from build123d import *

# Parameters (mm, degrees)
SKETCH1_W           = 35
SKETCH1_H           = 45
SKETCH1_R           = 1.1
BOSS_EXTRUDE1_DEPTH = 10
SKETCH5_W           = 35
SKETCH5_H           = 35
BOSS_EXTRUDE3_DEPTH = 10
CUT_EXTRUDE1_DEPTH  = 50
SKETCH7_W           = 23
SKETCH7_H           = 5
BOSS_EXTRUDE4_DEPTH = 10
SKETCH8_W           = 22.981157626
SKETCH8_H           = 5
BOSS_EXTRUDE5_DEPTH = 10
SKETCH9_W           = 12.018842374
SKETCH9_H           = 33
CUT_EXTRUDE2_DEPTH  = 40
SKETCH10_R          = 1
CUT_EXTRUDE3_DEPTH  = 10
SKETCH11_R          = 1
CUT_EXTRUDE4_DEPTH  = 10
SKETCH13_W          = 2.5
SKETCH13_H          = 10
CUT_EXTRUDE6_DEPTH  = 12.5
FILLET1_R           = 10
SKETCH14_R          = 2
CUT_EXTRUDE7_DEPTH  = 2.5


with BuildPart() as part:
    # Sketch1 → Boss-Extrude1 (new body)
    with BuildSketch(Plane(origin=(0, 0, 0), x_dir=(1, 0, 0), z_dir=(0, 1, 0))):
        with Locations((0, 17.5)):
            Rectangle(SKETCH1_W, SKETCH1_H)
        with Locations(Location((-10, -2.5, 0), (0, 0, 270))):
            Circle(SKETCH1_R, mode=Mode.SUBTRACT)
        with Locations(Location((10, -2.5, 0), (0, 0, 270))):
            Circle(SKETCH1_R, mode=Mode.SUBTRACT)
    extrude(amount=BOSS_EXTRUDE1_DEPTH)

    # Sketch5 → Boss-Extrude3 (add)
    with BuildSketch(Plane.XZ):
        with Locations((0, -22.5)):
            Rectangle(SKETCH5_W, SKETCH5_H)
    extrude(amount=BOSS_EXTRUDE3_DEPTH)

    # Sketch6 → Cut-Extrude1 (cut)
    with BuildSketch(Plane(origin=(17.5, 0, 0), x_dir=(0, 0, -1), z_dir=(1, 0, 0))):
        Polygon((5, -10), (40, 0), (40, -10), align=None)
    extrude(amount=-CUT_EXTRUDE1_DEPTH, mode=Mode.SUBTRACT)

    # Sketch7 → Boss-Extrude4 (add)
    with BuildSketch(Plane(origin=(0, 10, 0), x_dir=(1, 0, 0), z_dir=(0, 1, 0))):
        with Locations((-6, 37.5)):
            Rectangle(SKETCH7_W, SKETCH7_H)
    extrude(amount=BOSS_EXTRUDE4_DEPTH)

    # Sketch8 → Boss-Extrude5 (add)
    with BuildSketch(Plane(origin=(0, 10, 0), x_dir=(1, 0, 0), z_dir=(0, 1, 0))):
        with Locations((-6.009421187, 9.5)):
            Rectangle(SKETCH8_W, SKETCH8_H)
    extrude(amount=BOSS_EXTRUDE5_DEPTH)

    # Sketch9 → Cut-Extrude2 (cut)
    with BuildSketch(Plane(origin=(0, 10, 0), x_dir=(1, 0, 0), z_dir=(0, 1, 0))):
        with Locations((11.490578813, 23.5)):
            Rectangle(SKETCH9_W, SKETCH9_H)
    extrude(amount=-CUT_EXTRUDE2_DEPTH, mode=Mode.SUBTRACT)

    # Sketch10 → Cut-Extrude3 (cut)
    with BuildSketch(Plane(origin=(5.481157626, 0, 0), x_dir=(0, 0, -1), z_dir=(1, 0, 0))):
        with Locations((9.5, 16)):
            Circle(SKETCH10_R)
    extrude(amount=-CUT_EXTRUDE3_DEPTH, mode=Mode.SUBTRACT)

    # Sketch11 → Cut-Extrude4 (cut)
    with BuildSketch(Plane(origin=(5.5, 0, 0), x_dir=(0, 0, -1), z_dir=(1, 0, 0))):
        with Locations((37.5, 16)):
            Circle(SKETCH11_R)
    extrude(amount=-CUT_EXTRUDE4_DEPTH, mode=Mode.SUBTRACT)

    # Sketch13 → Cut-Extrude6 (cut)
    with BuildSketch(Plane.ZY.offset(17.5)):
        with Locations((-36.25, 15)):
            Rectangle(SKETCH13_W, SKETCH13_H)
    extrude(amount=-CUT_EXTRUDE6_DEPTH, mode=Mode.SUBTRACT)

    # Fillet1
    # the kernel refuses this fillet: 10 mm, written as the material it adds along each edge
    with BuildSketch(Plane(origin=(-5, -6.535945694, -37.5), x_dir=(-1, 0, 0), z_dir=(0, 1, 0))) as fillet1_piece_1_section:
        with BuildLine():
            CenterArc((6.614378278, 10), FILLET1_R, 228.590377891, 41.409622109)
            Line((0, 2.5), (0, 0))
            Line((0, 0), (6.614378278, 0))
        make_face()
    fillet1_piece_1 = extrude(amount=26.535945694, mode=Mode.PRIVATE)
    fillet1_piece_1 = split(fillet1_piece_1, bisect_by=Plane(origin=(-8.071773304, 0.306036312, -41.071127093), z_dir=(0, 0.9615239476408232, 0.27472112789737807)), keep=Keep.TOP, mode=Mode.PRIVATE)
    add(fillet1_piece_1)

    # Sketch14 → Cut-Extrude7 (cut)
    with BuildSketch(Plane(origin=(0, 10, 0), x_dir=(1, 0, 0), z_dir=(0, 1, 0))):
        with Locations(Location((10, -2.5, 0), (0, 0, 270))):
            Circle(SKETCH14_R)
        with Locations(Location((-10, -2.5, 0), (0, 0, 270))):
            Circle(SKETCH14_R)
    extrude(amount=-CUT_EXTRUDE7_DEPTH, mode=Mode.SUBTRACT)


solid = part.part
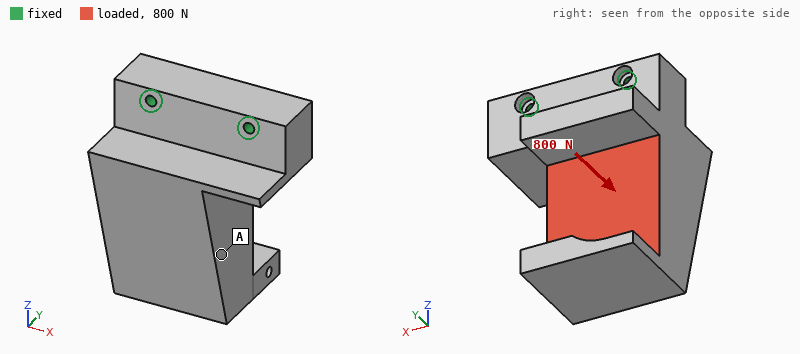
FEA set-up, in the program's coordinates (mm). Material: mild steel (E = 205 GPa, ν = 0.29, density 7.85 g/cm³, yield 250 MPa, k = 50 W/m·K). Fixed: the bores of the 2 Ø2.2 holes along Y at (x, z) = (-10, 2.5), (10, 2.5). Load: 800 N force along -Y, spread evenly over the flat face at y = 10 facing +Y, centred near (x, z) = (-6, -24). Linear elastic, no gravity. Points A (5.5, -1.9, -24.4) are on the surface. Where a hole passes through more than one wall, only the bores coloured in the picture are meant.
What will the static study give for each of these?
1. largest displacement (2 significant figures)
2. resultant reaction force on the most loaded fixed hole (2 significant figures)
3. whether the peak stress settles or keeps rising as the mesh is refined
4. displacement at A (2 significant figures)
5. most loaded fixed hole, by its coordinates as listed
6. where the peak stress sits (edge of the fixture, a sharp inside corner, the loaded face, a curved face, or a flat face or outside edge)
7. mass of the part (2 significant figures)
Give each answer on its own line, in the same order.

44 µm
580 N
keeps rising
24 µm
(-10, 2.5)
edge of the fixture
140 g
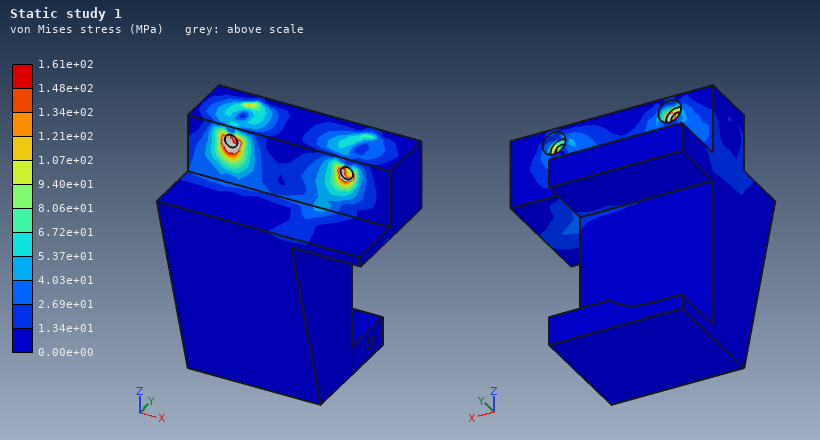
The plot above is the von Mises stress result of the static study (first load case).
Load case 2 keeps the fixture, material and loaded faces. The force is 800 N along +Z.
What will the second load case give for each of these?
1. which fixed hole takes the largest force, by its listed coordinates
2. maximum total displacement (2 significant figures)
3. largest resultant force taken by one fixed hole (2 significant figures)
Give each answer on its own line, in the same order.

(-10, 2.5)
12 µm
640 N
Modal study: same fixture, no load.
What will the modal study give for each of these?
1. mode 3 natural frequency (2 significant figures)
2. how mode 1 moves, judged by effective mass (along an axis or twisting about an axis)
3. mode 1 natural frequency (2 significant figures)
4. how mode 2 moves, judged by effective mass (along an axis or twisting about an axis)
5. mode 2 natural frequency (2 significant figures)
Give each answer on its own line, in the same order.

12 kHz
along Y
2800 Hz
along X
6700 Hz
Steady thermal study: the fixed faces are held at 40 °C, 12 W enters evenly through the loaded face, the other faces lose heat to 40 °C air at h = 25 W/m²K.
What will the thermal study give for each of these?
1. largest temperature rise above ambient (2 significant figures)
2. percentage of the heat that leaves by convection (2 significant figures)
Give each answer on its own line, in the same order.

22 K
14 %
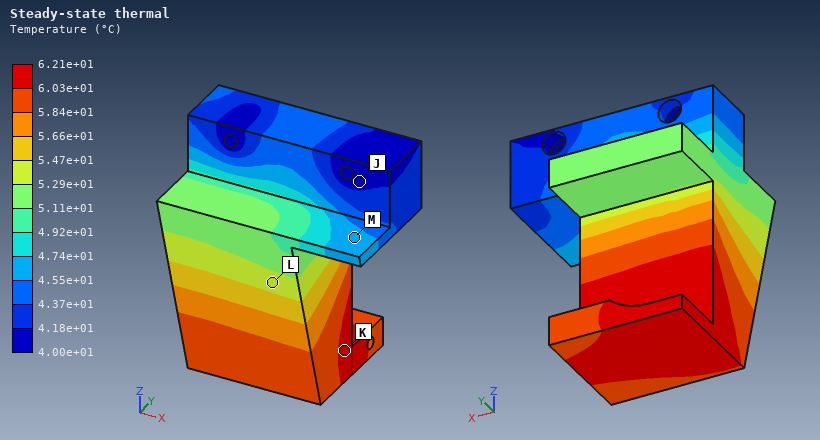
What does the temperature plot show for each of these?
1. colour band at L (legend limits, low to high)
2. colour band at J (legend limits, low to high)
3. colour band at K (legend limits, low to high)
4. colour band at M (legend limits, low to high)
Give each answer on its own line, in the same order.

5.29e+01 to 5.47e+01 °C
4.00e+01 to 4.18e+01 °C
6.03e+01 to 6.21e+01 °C
4.55e+01 to 4.74e+01 °C
